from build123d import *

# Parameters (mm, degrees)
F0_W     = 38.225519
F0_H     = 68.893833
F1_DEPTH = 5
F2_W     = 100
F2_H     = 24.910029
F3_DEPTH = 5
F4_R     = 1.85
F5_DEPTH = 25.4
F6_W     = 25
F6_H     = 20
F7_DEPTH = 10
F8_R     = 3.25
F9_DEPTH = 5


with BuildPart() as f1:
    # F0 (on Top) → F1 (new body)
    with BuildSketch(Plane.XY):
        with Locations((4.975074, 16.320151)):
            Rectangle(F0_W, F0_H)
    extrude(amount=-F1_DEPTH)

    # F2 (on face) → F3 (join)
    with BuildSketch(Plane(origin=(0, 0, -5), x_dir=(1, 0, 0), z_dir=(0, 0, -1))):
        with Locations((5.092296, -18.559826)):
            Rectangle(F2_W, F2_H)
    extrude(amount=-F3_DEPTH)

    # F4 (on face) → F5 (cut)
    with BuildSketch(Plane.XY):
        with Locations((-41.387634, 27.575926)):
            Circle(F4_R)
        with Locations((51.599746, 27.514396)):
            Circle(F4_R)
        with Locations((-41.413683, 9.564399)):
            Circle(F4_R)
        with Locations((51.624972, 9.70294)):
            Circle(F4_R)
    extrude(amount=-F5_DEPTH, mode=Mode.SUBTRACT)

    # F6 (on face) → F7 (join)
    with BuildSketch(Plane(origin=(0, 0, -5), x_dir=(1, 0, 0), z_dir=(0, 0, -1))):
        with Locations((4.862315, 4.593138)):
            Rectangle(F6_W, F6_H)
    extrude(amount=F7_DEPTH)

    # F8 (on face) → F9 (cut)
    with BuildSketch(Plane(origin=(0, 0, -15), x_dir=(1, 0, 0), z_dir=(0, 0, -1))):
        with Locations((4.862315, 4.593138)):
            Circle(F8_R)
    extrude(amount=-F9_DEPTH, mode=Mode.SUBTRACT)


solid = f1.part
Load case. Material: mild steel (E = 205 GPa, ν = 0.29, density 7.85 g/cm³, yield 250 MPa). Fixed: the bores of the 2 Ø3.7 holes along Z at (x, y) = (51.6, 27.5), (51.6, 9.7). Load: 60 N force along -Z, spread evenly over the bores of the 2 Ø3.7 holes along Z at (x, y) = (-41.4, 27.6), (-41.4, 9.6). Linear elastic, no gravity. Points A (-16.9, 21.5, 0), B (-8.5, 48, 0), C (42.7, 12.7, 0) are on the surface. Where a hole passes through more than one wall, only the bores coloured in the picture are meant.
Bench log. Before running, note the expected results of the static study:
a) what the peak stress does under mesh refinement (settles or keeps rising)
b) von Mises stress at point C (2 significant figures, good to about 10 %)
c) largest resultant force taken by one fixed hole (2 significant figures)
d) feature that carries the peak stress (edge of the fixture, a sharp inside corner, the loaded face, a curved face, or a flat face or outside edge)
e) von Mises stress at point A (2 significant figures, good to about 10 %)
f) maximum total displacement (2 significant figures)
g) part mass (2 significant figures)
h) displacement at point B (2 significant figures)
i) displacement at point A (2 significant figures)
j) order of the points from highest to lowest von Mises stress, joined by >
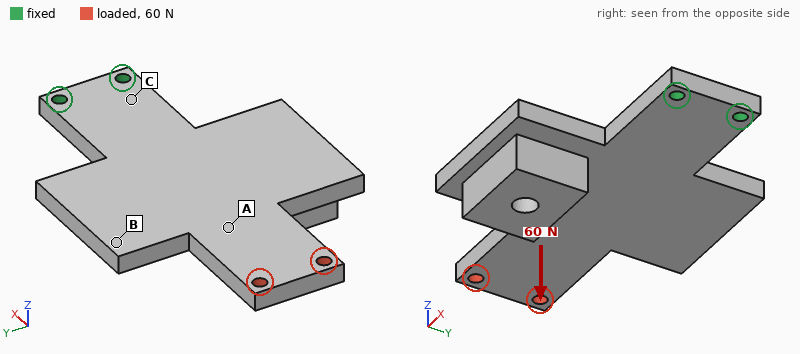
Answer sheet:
keeps rising
47 MPa
30 N
edge of the fixture
14 MPa
0.27 mm
200 g
0.13 mm
0.17 mm
C > A > B
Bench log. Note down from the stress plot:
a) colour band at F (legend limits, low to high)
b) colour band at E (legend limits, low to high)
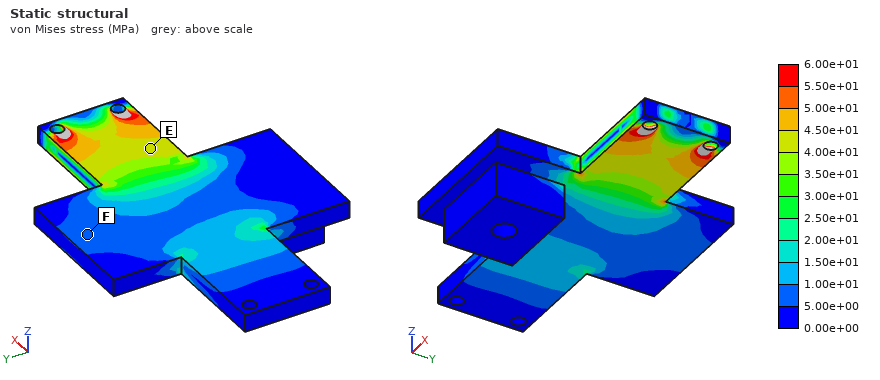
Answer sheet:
5.00e+00 to 1.00e+01 MPa
4.00e+01 to 4.50e+01 MPa
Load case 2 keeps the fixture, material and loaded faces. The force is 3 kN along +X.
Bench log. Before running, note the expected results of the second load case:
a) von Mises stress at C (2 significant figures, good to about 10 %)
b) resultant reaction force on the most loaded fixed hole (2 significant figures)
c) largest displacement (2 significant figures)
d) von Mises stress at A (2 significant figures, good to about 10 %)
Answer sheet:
25 MPa
1.5 kN
12 µm
20 MPa
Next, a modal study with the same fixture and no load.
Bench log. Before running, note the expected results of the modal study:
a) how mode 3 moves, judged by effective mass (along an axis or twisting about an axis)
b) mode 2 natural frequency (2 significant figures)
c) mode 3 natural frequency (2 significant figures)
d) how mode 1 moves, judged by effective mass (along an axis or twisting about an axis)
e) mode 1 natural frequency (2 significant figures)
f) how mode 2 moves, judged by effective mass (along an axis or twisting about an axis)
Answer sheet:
along Y
990 Hz
1600 Hz
along Z
370 Hz
twisting about X
